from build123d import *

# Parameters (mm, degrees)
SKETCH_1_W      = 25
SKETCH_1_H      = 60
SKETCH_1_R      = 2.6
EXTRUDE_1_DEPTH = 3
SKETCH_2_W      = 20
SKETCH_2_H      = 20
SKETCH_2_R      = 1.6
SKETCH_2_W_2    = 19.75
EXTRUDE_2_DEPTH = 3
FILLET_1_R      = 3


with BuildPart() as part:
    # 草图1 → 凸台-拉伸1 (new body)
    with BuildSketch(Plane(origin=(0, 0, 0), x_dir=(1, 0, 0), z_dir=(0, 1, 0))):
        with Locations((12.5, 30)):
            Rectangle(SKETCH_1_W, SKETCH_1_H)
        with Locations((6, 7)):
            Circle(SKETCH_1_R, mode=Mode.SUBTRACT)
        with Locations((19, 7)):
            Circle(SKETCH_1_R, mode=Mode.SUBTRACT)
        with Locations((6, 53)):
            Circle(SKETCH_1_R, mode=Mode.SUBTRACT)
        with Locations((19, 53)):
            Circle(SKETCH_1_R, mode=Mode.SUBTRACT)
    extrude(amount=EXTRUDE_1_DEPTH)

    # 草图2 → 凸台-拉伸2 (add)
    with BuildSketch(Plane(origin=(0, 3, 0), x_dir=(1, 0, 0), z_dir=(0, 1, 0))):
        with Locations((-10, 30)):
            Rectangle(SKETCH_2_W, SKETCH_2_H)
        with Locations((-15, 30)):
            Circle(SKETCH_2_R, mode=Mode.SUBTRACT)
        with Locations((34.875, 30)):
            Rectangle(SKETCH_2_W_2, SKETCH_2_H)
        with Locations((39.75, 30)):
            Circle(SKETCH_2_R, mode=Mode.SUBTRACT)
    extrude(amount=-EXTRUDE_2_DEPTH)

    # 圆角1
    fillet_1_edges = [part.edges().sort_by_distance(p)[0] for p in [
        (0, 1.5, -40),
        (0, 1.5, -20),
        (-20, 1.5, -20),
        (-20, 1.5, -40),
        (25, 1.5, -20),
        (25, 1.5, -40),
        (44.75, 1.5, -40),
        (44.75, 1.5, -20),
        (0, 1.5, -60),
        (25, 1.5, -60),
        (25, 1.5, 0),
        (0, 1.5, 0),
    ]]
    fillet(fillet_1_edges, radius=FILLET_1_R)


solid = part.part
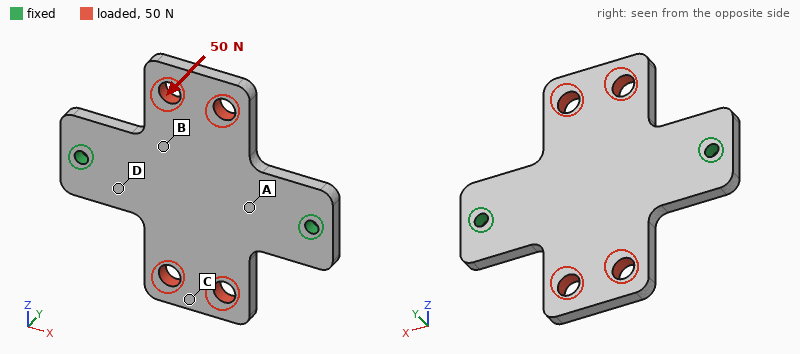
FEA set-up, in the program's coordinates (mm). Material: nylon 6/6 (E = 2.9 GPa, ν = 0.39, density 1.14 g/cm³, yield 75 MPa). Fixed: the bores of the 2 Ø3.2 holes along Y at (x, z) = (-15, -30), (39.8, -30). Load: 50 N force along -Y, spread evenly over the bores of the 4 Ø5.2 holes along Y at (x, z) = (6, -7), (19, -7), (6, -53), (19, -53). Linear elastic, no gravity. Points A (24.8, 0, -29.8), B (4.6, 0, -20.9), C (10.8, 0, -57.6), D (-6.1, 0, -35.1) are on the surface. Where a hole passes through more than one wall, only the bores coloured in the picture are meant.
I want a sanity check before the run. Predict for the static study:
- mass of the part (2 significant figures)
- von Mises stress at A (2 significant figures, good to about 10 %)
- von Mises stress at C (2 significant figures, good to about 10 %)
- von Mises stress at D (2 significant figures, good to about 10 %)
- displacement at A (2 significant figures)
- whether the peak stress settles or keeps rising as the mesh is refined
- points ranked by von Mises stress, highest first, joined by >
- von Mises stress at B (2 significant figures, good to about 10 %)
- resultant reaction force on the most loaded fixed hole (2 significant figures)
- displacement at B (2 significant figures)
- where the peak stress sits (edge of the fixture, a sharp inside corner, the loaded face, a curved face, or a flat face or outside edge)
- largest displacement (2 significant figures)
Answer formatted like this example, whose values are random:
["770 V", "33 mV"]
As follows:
["7.5 g", "6.7 MPa", "1.9 MPa", "4.5 MPa", "0.16 mm", "keeps rising", "B > A > D > C", "9.1 MPa", "25 N", "0.29 mm", "edge of the fixture", "0.93 mm"]
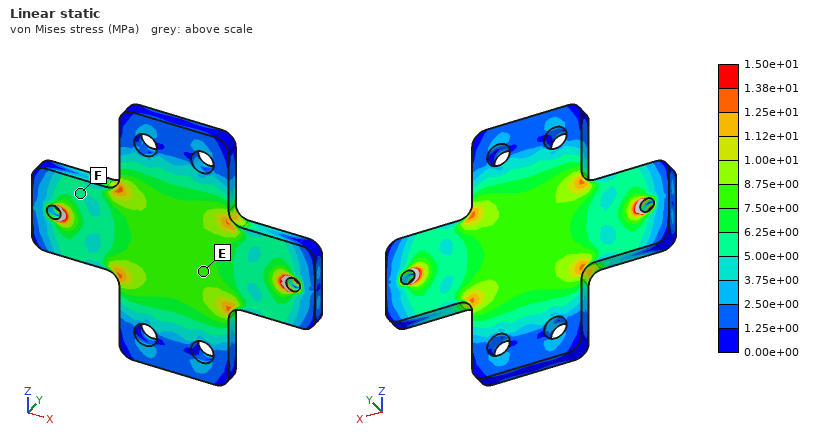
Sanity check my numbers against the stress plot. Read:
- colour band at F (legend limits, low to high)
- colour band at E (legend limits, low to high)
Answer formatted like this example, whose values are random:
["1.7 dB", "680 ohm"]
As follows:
["5.00e+00 to 6.25e+00 MPa", "7.50e+00 to 8.75e+00 MPa"]
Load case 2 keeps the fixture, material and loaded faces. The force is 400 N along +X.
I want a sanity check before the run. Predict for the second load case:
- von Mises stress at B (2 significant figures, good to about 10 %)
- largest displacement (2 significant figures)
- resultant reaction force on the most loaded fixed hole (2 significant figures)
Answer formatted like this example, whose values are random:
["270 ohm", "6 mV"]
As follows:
["3.5 MPa", "0.12 mm", "200 N"]
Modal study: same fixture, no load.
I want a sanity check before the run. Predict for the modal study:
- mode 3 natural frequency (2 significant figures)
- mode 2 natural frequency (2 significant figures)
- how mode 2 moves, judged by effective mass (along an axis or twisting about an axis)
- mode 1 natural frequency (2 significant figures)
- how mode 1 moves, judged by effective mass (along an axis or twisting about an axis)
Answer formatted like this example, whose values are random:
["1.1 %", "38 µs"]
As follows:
["2200 Hz", "810 Hz", "along Y", "580 Hz", "twisting about X"]
